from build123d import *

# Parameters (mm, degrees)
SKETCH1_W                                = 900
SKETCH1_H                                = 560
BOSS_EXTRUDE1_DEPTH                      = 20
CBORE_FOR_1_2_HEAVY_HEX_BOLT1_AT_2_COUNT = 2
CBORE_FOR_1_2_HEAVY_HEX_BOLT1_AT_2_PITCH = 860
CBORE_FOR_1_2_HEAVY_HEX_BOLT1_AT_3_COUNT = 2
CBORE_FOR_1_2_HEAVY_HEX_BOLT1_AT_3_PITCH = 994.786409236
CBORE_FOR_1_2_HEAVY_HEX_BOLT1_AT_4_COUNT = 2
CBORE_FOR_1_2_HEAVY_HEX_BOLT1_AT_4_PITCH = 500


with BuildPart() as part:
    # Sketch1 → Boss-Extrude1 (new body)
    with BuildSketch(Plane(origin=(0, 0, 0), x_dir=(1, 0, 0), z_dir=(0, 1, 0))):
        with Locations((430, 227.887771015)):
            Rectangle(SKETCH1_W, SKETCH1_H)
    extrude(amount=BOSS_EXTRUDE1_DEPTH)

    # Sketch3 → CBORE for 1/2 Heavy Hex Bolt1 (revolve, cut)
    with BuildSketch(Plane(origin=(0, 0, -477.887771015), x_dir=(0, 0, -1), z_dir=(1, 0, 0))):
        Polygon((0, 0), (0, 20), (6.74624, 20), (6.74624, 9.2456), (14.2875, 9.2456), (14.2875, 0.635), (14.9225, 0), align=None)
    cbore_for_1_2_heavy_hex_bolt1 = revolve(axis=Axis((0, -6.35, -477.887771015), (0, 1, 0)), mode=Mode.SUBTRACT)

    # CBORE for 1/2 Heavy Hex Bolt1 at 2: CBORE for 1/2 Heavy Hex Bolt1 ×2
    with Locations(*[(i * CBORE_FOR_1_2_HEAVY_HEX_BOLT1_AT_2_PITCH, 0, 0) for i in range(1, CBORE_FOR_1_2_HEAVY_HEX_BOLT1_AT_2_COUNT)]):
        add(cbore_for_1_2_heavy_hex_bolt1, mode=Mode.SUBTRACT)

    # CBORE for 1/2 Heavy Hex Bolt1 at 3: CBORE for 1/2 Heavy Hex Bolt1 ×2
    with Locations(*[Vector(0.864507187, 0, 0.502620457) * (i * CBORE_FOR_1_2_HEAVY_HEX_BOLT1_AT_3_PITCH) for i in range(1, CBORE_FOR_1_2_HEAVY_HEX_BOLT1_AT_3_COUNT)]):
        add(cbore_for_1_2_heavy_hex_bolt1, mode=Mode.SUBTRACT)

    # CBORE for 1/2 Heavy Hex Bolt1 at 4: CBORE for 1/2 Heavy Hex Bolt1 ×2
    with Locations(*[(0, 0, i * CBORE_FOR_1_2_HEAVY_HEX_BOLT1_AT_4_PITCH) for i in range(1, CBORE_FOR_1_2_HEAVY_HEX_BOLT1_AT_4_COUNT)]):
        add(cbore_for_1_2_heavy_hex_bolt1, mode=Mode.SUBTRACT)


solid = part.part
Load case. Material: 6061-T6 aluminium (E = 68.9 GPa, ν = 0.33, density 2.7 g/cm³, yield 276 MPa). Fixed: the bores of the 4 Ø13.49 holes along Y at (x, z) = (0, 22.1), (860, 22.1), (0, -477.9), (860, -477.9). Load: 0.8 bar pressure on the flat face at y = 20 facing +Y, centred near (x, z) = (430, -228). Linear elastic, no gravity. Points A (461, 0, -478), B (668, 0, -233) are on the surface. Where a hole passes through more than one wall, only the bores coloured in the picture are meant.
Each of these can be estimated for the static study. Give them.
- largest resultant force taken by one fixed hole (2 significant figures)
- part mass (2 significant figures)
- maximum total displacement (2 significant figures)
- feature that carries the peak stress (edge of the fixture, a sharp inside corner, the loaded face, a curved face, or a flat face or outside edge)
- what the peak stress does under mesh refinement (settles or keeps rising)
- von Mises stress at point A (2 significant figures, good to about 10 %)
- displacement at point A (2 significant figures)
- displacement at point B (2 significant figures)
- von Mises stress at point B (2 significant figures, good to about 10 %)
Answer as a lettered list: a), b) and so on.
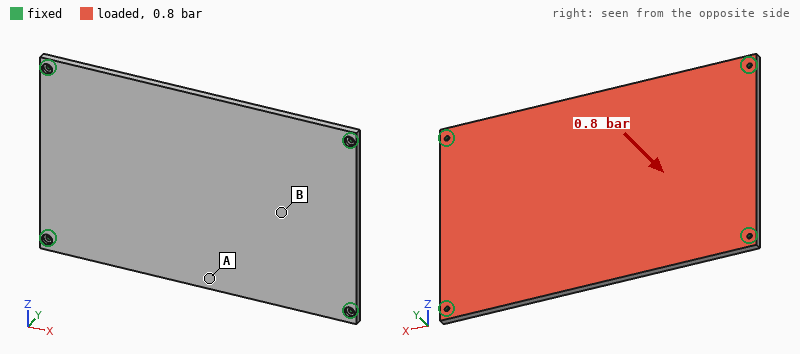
a) 28 kN
b) 27 kg
c) 5.8 mm
d) edge of the fixture
e) keeps rising
f) 68 MPa
g) 5.7 mm
h) 3.8 mm
i) 31 MPa
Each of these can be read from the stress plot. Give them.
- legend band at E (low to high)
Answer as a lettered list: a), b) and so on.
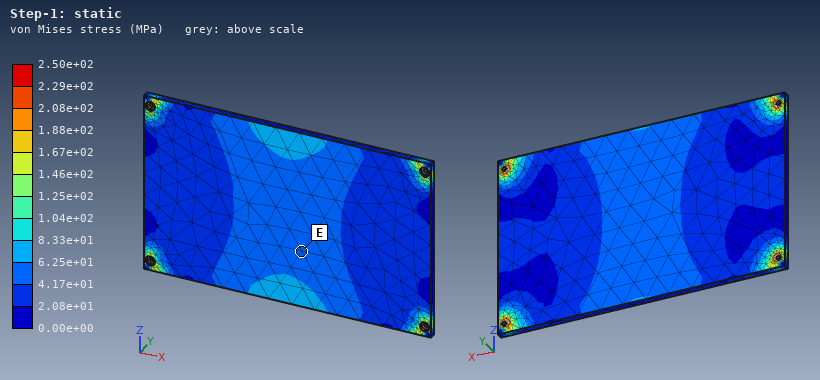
a) 4.17e+01 to 6.25e+01 MPa
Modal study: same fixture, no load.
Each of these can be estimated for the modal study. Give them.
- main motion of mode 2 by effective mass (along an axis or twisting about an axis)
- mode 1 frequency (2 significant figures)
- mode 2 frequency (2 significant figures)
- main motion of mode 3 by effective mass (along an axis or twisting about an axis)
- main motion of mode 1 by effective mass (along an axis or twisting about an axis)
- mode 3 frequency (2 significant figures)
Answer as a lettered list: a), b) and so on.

a) twisting about X
b) 92 Hz
c) 170 Hz
d) twisting about Z
e) along Y
f) 250 Hz
